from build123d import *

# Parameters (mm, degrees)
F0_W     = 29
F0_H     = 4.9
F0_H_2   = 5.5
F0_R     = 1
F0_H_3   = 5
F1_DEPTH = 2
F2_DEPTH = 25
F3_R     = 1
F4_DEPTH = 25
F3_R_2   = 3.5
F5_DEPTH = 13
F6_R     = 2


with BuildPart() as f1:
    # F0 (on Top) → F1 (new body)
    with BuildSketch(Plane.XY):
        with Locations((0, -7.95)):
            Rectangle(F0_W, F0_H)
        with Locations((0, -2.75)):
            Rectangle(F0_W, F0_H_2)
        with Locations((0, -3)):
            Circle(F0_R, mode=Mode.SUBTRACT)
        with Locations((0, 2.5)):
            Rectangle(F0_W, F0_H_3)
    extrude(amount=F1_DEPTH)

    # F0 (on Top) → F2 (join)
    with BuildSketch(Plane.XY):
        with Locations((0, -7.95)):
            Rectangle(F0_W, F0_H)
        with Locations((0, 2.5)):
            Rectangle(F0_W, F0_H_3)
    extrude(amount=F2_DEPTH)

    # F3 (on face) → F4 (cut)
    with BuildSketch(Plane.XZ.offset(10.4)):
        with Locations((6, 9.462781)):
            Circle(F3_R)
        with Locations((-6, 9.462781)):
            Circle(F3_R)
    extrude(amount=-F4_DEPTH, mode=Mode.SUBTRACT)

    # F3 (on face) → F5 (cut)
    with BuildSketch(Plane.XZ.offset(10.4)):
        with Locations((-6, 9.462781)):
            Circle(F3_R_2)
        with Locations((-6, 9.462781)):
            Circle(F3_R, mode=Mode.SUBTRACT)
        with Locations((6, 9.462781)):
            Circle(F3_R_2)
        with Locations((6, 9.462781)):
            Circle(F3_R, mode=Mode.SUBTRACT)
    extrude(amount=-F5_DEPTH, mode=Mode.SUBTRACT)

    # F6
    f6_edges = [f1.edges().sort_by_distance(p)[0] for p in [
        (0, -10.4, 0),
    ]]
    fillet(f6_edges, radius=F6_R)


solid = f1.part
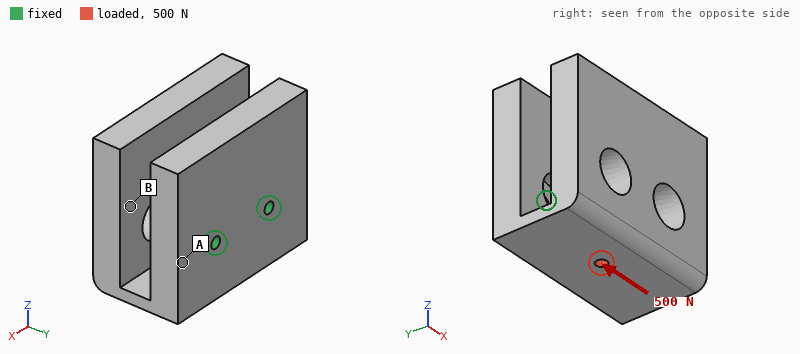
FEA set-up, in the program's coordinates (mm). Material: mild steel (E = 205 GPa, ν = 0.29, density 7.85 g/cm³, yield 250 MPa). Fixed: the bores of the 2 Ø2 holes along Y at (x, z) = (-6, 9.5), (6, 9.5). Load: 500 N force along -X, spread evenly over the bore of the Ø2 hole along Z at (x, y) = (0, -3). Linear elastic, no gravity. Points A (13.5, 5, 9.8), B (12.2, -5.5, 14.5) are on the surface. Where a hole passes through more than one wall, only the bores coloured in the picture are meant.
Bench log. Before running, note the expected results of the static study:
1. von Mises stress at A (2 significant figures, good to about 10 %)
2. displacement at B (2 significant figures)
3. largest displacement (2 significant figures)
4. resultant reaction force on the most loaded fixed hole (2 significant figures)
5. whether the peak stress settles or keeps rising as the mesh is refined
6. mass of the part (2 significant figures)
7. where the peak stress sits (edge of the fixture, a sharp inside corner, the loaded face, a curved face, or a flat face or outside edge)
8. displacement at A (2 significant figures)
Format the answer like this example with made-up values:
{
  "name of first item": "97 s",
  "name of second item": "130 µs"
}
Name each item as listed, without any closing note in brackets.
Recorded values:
{
  "von Mises stress at A": "14 MPa",
  "displacement at B": "5.9 µm",
  "largest displacement": "7.9 µm",
  "resultant reaction force on the most loaded fixed hole": "480 N",
  "whether the peak stress settles or keeps rising as the mesh is refined": "keeps rising",
  "mass of the part": "54 g",
  "where the peak stress sits": "edge of the fixture",
  "displacement at A": "2.0 µm"
}
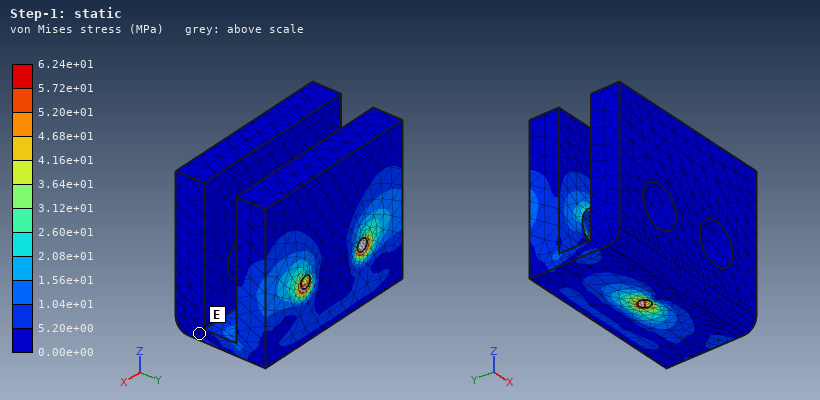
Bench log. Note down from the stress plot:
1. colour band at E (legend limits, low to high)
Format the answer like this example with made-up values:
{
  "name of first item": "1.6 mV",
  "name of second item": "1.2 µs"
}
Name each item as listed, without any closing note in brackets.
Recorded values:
{
  "colour band at E": "0.00e+00 to 5.20e+00 MPa"
}
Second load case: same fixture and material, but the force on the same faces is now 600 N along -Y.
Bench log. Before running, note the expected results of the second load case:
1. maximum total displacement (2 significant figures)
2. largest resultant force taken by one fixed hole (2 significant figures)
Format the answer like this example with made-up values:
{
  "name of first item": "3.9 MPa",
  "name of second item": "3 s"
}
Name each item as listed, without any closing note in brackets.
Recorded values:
{
  "maximum total displacement": "38 µm",
  "largest resultant force taken by one fixed hole": "300 N"
}
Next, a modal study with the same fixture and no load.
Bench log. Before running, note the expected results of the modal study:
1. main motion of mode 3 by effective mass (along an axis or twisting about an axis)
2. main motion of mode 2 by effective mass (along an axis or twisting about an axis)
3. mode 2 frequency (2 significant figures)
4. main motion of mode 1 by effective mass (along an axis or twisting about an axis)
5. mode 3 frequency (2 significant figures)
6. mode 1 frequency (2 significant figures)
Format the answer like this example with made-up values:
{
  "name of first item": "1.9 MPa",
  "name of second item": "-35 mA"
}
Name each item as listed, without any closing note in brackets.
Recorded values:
{
  "main motion of mode 3 by effective mass": "along Z",
  "main motion of mode 2 by effective mass": "along X",
  "mode 2 frequency": "3400 Hz",
  "main motion of mode 1 by effective mass": "along Y",
  "mode 3 frequency": "4300 Hz",
  "mode 1 frequency": "1400 Hz"
}
